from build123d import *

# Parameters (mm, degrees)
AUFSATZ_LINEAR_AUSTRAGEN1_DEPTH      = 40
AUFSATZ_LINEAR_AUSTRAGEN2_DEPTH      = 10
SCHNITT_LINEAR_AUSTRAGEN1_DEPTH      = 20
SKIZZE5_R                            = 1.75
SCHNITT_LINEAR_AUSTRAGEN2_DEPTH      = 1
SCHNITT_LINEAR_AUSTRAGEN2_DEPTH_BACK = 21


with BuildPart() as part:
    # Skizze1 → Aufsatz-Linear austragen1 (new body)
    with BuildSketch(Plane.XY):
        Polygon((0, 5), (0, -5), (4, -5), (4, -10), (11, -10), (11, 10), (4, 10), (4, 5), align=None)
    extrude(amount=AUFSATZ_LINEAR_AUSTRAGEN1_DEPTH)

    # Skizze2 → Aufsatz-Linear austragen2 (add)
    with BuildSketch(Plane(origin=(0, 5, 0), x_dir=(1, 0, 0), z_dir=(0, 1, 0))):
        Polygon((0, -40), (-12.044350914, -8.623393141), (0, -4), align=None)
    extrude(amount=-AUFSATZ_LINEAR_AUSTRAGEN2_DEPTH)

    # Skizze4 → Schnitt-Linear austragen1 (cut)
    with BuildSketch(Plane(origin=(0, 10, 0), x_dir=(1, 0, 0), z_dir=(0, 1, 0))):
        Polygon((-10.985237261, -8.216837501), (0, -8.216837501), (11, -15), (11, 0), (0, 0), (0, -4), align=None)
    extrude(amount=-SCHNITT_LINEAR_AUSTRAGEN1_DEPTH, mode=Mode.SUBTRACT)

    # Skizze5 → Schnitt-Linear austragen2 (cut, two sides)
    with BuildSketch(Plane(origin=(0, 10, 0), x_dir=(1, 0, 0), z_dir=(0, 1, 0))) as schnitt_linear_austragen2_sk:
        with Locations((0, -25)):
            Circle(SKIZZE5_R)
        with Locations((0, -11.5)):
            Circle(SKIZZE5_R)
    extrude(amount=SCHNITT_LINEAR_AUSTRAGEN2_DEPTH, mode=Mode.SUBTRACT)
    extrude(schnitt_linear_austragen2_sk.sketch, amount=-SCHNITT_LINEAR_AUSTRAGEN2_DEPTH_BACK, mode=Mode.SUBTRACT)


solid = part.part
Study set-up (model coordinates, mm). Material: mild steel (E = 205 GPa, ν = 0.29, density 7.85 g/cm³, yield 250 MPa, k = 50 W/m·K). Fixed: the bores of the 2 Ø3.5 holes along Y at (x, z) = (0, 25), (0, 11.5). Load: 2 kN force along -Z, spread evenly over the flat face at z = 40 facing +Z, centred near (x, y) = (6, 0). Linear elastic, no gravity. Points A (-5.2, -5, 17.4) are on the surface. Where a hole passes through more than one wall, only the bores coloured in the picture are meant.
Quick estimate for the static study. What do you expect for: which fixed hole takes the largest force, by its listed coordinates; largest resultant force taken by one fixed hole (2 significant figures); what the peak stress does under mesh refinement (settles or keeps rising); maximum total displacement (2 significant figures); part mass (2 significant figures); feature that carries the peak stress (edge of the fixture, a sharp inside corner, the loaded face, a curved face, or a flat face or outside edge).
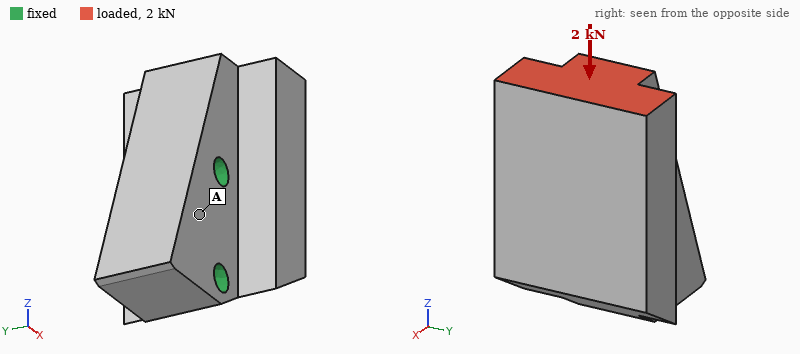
(0, 25)
1.5 kN
keeps rising
3.1 µm
53 g
edge of the fixture
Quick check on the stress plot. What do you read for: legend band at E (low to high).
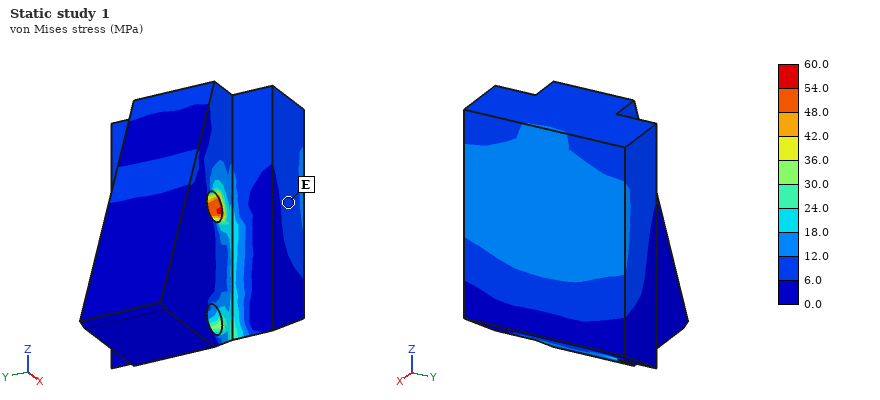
6.0 to 12.0 MPa
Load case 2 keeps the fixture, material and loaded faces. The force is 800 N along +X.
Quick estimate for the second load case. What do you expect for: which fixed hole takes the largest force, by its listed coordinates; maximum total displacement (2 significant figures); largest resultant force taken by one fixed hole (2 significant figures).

(0, 25)
4.3 µm
1.5 kN
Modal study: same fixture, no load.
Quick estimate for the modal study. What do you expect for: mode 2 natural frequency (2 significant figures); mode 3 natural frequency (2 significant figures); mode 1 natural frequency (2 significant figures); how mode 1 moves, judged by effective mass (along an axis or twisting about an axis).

24 kHz
29 kHz
20 kHz
along Y
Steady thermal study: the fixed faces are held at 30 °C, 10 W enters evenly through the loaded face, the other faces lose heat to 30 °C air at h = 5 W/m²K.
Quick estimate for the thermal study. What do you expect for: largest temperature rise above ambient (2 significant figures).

19 K
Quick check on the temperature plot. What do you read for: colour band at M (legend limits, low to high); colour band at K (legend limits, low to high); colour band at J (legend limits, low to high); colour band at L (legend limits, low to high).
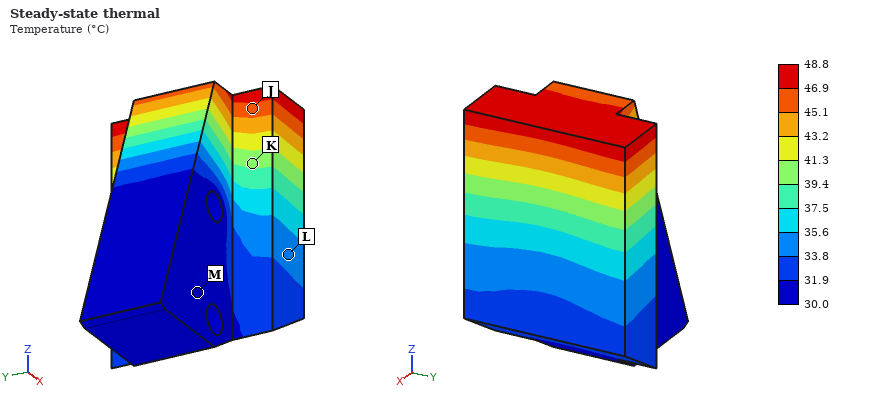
30.0 to 31.9 °C
39.4 to 41.3 °C
45.1 to 46.9 °C
33.8 to 35.6 °C
